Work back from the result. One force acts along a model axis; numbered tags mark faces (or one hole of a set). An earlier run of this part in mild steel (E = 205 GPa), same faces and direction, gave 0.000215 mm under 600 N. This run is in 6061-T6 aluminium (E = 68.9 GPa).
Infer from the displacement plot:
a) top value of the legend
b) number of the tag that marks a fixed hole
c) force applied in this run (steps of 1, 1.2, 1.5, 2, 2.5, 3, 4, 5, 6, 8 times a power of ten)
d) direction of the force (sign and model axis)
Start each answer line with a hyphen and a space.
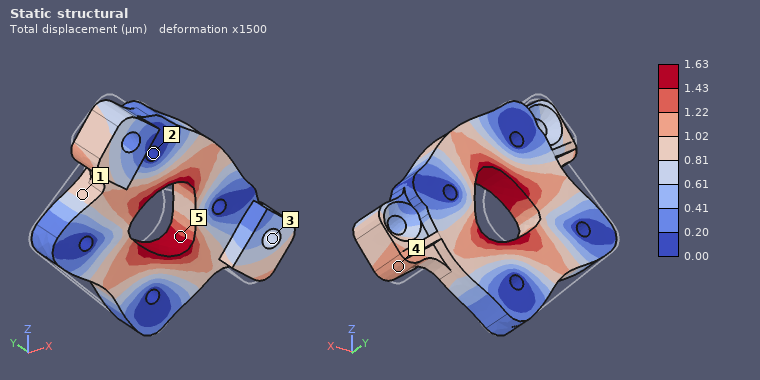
- 1.63 µm
- 2
- 1.5 kN
- +X
